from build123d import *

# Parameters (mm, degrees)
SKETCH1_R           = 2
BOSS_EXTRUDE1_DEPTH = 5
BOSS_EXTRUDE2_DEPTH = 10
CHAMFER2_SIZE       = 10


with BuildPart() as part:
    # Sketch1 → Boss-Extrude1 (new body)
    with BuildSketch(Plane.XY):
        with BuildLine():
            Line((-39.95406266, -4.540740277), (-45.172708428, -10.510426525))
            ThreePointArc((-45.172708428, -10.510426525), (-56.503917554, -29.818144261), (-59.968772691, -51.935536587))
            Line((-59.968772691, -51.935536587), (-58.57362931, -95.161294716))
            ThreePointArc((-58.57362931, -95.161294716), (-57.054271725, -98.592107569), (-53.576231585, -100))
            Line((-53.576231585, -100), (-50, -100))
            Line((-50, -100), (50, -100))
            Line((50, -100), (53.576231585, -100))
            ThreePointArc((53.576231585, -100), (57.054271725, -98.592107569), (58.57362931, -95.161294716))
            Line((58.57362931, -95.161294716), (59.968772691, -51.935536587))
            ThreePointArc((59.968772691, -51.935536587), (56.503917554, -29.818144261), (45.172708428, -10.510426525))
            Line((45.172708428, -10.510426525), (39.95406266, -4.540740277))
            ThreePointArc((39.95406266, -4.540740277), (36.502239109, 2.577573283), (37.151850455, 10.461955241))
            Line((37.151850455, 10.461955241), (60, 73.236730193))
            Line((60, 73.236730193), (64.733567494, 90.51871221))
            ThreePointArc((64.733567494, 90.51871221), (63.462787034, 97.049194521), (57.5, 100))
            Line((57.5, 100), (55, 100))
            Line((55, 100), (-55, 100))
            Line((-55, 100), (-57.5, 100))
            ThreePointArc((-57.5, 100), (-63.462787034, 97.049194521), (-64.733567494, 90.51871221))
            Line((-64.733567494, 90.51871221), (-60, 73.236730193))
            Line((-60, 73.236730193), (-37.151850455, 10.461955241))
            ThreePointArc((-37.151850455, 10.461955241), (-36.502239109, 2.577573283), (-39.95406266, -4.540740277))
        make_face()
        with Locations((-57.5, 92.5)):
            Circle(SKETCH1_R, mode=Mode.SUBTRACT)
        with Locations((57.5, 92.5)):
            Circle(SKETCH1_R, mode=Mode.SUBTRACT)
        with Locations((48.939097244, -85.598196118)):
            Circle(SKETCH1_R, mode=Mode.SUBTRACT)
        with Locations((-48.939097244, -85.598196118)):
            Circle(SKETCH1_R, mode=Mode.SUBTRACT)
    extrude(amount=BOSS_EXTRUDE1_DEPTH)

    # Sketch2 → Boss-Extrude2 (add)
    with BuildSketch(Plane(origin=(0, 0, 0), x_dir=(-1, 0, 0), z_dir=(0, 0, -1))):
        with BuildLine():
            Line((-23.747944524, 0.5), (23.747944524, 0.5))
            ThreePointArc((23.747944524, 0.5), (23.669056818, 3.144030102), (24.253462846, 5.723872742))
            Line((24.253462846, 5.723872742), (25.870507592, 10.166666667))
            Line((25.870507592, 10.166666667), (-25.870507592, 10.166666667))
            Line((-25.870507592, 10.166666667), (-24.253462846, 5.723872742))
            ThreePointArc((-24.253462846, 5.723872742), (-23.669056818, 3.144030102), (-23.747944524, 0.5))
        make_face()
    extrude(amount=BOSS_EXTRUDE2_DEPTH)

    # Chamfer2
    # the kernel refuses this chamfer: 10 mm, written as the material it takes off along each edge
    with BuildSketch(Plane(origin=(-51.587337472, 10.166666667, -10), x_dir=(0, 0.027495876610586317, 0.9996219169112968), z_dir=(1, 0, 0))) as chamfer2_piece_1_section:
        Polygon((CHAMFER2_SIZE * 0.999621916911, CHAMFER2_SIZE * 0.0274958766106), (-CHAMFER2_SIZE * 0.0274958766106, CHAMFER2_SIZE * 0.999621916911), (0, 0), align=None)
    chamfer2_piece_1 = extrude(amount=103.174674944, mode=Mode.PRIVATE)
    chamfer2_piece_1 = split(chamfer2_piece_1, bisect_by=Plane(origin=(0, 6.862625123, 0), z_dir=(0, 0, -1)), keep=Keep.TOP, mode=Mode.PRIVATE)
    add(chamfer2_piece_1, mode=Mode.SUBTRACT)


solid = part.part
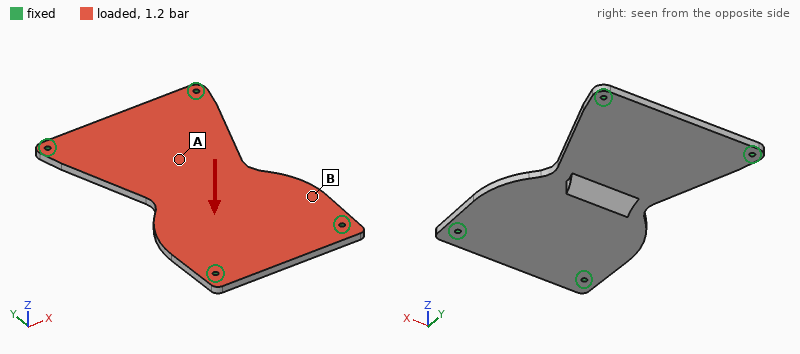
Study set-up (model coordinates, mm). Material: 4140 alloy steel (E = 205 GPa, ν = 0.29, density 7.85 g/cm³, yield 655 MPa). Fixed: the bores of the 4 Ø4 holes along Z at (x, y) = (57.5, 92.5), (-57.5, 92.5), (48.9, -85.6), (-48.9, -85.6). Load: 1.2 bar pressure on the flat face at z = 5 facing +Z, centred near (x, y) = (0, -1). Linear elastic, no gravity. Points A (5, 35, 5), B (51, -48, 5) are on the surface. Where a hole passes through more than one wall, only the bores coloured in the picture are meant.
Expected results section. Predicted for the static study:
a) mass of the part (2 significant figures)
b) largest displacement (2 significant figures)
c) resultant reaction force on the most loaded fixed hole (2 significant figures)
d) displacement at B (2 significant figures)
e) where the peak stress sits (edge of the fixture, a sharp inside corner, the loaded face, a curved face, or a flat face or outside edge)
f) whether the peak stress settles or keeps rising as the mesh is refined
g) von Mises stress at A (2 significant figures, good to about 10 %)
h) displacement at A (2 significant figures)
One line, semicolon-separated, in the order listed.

850 g; 0.24 mm; 690 N; 0.10 mm; edge of the fixture; keeps rising; 33 MPa; 0.21 mm
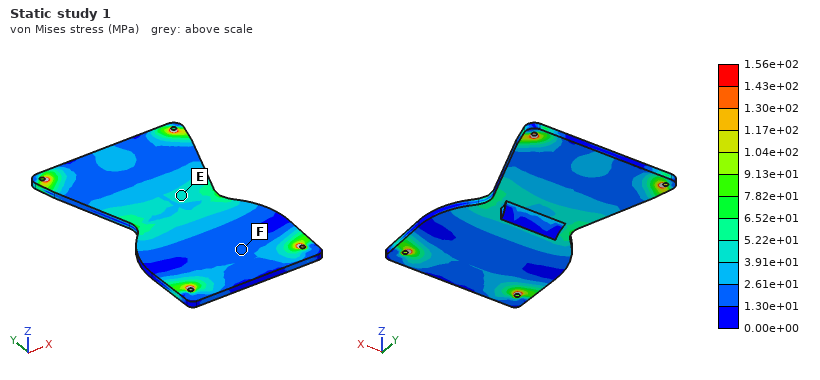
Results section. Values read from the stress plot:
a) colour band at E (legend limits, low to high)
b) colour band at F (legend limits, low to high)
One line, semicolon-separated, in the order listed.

3.91e+01 to 5.22e+01 MPa; 1.30e+01 to 2.61e+01 MPa
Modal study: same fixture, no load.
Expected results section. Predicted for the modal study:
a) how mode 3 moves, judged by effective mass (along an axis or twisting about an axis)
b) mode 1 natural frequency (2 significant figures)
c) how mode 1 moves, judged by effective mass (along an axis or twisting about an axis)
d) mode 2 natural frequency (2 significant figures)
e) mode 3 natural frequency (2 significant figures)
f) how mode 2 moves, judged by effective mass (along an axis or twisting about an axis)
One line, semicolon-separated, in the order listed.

twisting about X; 640 Hz; along Z; 1400 Hz; 1600 Hz; twisting about Y
